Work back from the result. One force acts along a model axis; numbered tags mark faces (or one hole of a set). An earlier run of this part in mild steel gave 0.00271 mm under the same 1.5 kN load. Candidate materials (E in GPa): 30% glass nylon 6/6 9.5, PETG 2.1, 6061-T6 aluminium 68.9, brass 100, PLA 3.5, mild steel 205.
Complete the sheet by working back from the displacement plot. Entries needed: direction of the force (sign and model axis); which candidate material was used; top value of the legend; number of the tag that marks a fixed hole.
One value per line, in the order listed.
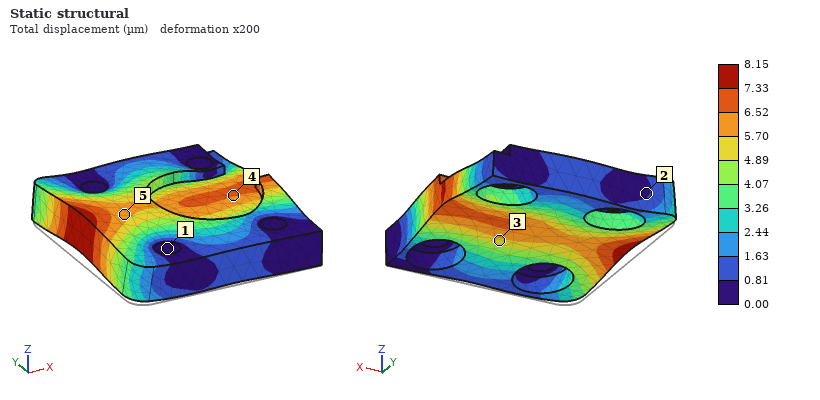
+Z
6061-T6 aluminium
8.15 µm
1
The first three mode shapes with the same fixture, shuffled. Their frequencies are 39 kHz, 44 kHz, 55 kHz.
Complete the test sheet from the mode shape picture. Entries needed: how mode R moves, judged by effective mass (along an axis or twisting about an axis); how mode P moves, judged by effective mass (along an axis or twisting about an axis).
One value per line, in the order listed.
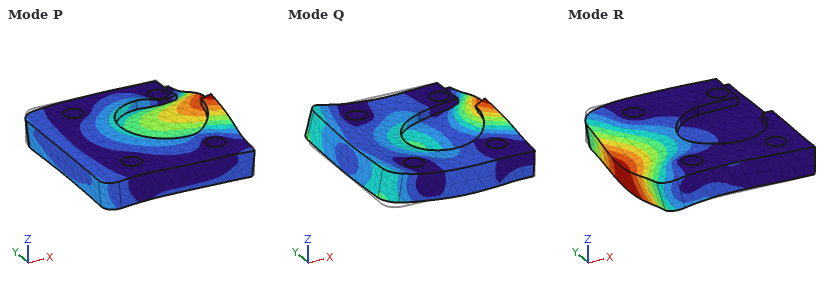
along Z
along Z
